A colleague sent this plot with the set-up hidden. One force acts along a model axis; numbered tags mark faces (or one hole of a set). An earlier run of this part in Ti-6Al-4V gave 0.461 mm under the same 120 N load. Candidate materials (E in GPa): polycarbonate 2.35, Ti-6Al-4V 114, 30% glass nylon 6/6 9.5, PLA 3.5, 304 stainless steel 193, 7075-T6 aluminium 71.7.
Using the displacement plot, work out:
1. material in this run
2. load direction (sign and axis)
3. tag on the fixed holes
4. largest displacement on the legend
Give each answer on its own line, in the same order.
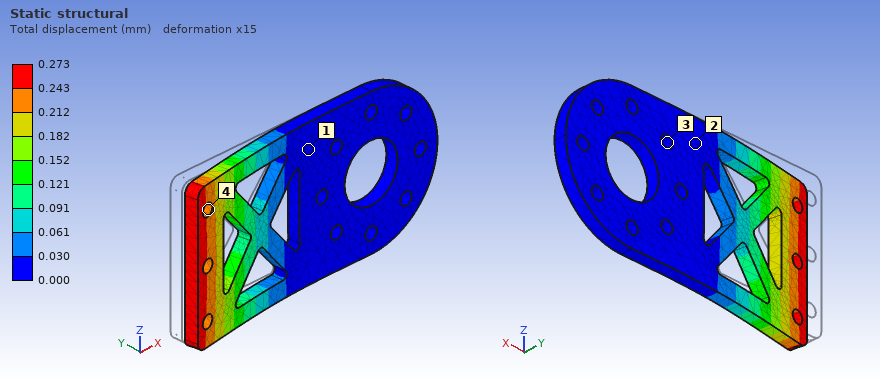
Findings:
304 stainless steel
-Y
3
0.273 mm
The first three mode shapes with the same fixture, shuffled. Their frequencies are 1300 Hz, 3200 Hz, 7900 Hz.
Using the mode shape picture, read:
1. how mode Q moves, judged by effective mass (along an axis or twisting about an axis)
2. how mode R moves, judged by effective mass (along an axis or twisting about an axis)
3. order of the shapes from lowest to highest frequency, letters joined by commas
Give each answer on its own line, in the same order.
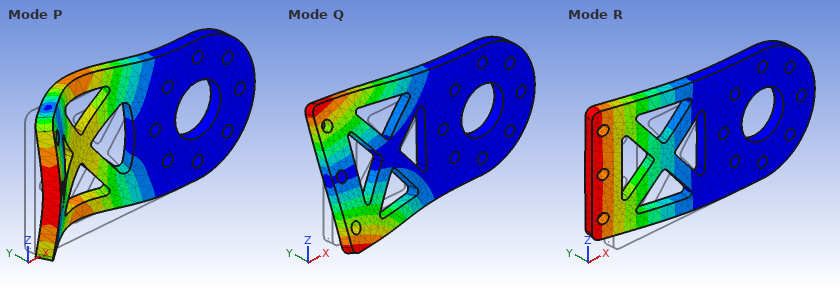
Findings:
twisting about X
along Y
R, Q, P
